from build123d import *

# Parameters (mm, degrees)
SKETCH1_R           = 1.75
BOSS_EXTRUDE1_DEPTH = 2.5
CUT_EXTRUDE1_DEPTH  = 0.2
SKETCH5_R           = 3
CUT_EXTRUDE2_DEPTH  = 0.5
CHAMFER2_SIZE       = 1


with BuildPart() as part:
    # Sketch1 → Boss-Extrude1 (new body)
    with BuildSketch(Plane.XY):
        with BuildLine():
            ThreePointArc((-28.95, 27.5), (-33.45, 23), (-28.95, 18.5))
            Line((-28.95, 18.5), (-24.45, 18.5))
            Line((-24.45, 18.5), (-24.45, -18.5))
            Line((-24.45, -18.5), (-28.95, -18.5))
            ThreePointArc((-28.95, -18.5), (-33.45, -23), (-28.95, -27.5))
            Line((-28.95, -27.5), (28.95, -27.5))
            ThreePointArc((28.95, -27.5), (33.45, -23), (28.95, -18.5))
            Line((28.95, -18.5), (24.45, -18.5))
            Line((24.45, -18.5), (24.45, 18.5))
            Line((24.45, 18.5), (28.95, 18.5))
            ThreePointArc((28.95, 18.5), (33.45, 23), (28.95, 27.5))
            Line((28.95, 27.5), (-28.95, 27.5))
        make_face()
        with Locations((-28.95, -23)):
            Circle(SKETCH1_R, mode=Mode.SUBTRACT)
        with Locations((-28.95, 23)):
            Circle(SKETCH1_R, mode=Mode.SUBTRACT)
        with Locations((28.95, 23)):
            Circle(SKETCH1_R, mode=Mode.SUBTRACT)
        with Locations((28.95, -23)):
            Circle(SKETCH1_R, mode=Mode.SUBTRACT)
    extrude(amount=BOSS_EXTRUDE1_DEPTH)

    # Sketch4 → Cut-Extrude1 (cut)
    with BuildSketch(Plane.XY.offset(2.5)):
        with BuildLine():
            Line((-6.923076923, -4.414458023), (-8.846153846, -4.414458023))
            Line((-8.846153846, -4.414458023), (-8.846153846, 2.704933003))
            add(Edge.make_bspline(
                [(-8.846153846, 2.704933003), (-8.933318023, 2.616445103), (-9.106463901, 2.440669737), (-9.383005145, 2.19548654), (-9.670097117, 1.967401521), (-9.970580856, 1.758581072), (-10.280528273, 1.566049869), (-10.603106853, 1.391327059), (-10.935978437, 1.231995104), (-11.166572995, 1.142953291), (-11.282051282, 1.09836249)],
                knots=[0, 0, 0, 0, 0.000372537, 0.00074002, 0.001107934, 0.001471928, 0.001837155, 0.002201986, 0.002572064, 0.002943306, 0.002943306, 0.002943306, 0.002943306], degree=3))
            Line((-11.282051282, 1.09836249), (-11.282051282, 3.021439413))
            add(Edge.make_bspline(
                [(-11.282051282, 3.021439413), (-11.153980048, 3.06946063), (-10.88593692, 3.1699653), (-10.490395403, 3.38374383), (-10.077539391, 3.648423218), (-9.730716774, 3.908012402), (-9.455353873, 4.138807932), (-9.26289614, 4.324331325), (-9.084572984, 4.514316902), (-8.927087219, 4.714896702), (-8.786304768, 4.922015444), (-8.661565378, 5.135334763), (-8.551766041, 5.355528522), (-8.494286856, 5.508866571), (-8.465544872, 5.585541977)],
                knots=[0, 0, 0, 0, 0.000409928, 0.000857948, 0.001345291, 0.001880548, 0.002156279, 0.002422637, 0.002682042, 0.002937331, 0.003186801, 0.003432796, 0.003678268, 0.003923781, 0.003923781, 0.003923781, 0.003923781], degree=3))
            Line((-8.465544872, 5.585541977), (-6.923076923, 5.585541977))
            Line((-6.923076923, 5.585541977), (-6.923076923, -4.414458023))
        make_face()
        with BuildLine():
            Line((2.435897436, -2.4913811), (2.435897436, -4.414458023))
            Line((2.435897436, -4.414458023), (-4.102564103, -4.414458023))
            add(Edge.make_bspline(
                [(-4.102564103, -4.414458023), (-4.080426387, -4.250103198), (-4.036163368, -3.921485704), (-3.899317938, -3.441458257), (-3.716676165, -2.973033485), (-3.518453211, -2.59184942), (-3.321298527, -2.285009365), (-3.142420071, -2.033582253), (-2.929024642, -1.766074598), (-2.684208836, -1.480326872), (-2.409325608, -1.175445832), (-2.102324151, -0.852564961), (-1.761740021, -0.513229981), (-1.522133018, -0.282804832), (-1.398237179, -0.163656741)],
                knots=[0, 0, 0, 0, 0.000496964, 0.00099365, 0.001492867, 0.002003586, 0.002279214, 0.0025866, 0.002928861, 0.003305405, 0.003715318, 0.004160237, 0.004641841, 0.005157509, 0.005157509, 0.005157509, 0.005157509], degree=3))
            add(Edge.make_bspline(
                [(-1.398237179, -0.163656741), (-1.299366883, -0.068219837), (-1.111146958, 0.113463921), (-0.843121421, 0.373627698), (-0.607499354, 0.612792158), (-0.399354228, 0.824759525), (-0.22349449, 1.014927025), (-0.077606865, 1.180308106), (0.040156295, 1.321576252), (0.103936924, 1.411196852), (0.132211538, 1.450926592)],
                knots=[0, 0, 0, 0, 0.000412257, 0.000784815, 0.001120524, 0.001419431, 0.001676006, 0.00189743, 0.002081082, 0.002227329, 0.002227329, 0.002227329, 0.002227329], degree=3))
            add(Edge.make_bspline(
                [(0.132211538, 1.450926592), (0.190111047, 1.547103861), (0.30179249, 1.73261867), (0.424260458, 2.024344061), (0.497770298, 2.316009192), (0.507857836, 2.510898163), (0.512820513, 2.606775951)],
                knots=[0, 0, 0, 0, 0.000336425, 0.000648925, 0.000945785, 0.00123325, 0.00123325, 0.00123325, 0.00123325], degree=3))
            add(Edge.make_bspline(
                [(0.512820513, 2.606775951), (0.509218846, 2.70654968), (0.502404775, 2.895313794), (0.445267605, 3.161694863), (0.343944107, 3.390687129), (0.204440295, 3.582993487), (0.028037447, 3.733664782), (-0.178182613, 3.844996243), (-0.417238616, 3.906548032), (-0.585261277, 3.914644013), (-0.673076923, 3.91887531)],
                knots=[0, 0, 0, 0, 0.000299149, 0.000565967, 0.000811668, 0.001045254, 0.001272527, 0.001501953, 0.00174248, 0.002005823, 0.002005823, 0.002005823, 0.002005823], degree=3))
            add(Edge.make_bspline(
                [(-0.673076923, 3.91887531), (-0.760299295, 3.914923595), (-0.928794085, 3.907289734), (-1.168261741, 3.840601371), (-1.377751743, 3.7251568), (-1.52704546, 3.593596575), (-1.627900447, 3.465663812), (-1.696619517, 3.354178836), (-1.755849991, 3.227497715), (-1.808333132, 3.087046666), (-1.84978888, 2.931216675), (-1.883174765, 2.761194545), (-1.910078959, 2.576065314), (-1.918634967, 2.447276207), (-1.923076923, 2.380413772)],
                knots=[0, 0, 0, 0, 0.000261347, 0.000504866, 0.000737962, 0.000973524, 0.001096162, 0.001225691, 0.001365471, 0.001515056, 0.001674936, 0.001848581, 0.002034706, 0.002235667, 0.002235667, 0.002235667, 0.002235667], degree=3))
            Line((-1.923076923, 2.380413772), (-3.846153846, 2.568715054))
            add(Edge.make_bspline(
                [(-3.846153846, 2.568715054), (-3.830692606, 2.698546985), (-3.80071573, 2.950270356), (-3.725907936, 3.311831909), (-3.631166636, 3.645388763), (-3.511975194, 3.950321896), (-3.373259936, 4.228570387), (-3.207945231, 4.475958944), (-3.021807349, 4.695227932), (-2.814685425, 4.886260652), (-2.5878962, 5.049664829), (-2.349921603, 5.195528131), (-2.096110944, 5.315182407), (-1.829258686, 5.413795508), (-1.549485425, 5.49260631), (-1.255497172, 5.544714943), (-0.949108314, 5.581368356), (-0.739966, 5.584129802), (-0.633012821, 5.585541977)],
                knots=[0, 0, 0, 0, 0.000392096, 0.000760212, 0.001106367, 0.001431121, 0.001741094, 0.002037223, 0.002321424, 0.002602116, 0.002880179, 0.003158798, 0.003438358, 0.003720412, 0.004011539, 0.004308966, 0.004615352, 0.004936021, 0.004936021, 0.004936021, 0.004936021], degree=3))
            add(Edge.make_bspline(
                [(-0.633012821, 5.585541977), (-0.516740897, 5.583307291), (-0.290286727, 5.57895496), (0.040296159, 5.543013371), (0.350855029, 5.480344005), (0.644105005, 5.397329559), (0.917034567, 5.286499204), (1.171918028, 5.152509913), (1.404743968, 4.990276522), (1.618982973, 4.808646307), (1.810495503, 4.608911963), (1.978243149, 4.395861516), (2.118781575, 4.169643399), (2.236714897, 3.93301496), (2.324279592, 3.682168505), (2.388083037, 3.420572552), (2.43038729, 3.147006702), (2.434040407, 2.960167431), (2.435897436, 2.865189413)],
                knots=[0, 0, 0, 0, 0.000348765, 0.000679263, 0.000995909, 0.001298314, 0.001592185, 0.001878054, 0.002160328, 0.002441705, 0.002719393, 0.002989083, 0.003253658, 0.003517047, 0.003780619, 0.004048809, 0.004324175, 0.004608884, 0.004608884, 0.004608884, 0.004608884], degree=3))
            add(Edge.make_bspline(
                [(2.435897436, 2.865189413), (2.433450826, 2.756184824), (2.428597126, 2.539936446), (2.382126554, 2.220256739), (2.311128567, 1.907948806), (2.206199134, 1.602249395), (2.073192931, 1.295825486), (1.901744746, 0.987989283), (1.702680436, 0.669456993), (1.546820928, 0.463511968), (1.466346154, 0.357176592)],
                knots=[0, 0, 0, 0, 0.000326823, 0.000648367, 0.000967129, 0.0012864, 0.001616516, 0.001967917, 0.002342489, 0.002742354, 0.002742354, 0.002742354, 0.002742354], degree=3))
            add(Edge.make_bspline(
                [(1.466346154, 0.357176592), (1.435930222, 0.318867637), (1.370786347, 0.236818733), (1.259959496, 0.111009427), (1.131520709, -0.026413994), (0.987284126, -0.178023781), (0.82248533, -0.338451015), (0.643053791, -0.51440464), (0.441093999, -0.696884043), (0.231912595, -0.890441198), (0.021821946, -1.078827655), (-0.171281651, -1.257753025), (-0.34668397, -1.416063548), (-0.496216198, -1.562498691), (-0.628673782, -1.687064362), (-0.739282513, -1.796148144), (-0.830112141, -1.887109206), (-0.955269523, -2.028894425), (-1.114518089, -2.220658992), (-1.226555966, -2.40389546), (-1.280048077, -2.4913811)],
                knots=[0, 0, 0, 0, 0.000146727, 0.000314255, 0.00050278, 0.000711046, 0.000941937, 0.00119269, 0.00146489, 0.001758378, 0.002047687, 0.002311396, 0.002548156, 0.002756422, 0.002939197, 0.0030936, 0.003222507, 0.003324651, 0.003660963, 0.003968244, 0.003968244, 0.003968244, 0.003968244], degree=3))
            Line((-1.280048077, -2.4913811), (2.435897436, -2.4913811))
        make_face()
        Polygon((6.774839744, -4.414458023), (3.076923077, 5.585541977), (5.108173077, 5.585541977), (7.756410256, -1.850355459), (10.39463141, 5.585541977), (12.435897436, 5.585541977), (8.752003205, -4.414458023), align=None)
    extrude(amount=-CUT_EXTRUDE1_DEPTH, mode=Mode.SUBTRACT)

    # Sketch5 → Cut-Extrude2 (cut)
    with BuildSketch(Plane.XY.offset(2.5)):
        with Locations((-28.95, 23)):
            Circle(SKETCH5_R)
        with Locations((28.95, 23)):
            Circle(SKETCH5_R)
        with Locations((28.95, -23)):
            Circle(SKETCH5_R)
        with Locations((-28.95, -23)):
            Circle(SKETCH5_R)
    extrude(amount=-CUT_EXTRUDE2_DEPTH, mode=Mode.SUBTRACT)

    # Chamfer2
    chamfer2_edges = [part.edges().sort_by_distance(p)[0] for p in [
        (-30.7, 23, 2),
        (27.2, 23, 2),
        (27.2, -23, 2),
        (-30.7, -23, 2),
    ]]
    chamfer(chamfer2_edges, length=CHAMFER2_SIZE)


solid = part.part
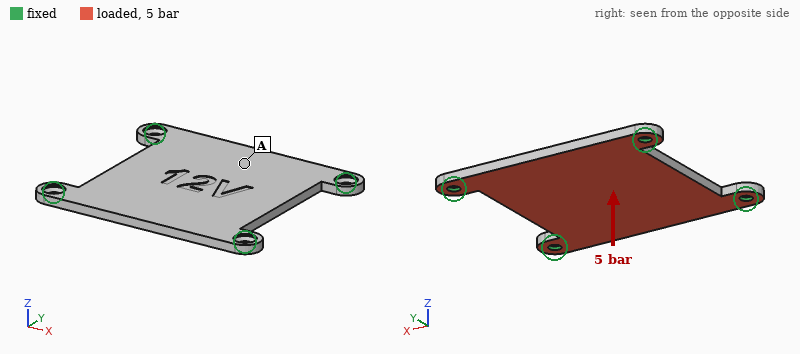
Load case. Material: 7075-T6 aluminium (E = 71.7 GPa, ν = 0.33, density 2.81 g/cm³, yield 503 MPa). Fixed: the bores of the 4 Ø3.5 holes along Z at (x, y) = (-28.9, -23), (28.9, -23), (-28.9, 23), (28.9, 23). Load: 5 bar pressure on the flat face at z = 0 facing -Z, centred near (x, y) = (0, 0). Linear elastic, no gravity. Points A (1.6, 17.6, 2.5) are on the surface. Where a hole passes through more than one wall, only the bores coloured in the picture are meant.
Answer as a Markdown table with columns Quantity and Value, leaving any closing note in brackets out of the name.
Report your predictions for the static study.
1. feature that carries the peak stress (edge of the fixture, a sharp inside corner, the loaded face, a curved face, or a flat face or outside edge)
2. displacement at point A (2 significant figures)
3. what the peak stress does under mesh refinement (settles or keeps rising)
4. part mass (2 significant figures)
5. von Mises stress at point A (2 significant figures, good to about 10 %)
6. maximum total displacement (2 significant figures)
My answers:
| Quantity | Value |
|---|---|
| feature that carries the peak stress | edge of the fixture |
| displacement at point A | 0.34 mm |
| what the peak stress does under mesh refinement | keeps rising |
| part mass | 20 g |
| von Mises stress at point A | 110 MPa |
| maximum total displacement | 0.40 mm |
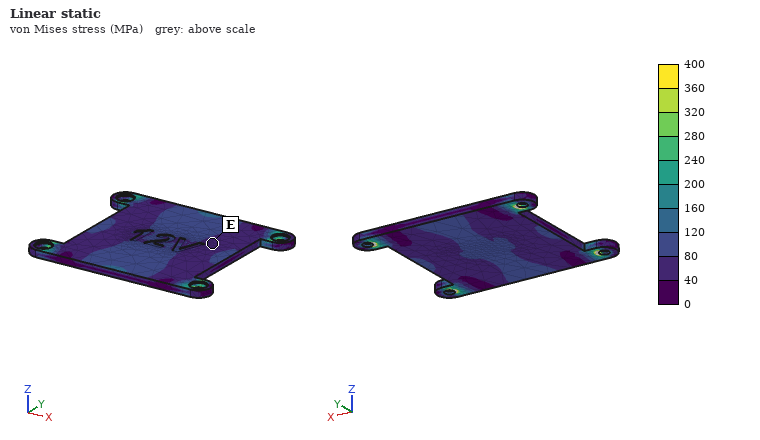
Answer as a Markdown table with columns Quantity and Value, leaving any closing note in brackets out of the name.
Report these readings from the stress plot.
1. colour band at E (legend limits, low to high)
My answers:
| Quantity | Value |
|---|---|
| colour band at E | 40 to 80 MPa |
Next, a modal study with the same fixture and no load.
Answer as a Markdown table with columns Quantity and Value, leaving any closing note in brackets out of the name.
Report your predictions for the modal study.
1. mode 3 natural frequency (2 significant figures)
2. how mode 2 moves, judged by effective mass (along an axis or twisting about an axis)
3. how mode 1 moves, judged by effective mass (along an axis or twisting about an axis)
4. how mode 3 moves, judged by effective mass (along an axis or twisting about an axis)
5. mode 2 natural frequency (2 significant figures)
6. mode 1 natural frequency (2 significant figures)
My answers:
| Quantity | Value |
|---|---|
| mode 3 natural frequency | 5400 Hz |
| how mode 2 moves, judged by effective mass | twisting about X |
| how mode 1 moves, judged by effective mass | along Z |
| how mode 3 moves, judged by effective mass | twisting about Y |
| mode 2 natural frequency | 4000 Hz |
| mode 1 natural frequency | 2500 Hz |
